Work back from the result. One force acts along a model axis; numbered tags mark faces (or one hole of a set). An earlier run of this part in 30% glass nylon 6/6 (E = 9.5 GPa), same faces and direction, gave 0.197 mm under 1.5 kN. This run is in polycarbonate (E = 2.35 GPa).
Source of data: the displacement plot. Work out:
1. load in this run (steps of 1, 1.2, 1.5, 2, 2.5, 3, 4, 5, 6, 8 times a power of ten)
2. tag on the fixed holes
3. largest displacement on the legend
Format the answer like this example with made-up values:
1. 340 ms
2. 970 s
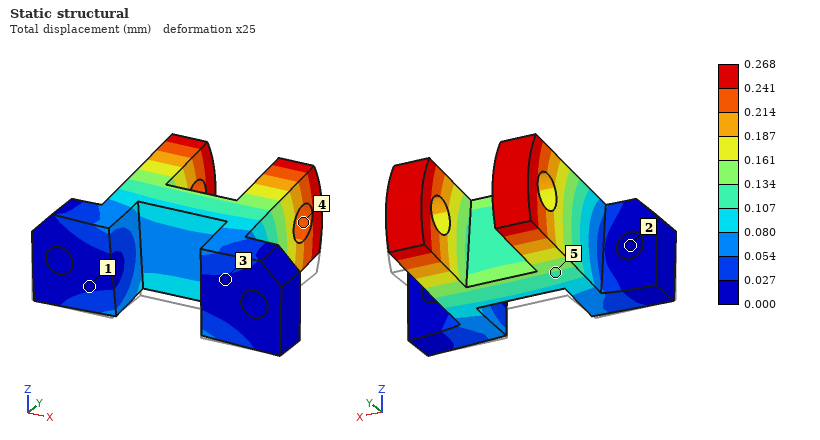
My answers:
1. 500 N
2. 2
3. 0.268 mm
